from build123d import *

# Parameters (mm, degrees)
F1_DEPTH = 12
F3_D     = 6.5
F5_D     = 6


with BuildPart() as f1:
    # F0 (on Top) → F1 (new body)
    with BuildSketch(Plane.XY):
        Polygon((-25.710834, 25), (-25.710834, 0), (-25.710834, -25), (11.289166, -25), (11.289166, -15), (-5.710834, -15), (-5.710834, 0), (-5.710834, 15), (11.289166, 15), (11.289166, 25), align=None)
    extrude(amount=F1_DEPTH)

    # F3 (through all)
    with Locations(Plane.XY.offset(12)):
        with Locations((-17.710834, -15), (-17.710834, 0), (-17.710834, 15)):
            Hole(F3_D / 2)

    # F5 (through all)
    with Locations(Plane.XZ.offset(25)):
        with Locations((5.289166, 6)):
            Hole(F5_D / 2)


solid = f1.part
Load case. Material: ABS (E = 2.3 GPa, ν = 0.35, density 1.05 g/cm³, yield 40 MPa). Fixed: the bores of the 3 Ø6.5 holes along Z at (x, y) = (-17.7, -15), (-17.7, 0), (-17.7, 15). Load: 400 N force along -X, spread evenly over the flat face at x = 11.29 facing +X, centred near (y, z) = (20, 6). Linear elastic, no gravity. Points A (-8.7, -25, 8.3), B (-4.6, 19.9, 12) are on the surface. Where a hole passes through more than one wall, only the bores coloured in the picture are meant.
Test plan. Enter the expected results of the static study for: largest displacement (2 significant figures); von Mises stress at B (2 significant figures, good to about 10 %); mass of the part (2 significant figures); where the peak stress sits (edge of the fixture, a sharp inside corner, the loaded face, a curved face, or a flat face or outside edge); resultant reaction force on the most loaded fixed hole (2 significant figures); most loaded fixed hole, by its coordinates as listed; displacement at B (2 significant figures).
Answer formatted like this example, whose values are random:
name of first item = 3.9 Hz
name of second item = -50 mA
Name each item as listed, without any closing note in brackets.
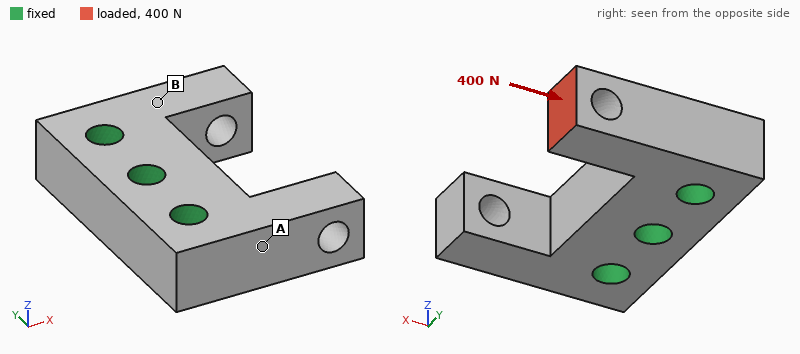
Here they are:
largest displacement = 99 µm
von Mises stress at B = 4.1 MPa
mass of the part = 15 g
where the peak stress sits = a curved face
resultant reaction force on the most loaded fixed hole = 440 N
most loaded fixed hole, by its coordinates as listed = (-17.7, 15)
displacement at B = 28 µm
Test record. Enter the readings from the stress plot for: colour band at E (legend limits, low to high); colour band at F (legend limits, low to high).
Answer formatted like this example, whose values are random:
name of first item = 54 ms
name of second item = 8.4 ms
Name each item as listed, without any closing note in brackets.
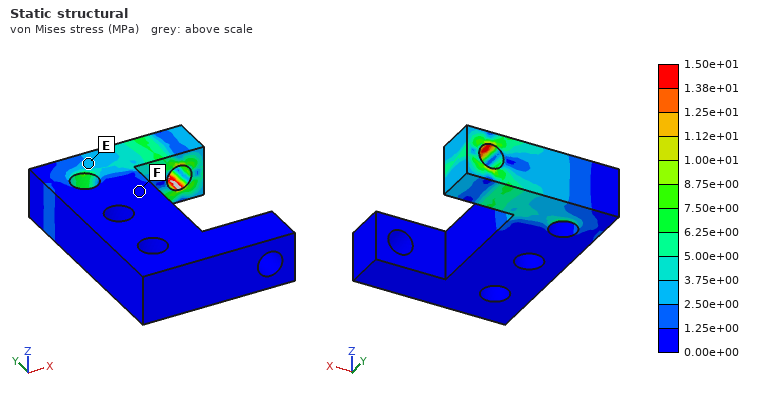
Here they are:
colour band at E = 2.50e+00 to 3.75e+00 MPa
colour band at F = 0.00e+00 to 1.25e+00 MPa
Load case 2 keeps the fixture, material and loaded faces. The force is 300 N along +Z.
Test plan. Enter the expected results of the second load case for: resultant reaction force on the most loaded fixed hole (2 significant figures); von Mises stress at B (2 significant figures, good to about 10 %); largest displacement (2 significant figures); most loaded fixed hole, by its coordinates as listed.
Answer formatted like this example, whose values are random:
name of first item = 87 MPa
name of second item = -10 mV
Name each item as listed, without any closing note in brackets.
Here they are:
resultant reaction force on the most loaded fixed hole = 280 N
von Mises stress at B = 19 MPa
largest displacement = 0.73 mm
most loaded fixed hole, by its coordinates as listed = (-17.7, 15)
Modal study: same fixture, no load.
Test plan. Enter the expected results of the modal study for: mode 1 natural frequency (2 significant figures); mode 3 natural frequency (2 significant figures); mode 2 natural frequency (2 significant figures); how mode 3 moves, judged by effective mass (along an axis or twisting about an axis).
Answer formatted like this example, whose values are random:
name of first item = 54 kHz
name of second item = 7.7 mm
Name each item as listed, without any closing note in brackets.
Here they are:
mode 1 natural frequency = 3900 Hz
mode 3 natural frequency = 4300 Hz
mode 2 natural frequency = 3900 Hz
how mode 3 moves, judged by effective mass = along Y
